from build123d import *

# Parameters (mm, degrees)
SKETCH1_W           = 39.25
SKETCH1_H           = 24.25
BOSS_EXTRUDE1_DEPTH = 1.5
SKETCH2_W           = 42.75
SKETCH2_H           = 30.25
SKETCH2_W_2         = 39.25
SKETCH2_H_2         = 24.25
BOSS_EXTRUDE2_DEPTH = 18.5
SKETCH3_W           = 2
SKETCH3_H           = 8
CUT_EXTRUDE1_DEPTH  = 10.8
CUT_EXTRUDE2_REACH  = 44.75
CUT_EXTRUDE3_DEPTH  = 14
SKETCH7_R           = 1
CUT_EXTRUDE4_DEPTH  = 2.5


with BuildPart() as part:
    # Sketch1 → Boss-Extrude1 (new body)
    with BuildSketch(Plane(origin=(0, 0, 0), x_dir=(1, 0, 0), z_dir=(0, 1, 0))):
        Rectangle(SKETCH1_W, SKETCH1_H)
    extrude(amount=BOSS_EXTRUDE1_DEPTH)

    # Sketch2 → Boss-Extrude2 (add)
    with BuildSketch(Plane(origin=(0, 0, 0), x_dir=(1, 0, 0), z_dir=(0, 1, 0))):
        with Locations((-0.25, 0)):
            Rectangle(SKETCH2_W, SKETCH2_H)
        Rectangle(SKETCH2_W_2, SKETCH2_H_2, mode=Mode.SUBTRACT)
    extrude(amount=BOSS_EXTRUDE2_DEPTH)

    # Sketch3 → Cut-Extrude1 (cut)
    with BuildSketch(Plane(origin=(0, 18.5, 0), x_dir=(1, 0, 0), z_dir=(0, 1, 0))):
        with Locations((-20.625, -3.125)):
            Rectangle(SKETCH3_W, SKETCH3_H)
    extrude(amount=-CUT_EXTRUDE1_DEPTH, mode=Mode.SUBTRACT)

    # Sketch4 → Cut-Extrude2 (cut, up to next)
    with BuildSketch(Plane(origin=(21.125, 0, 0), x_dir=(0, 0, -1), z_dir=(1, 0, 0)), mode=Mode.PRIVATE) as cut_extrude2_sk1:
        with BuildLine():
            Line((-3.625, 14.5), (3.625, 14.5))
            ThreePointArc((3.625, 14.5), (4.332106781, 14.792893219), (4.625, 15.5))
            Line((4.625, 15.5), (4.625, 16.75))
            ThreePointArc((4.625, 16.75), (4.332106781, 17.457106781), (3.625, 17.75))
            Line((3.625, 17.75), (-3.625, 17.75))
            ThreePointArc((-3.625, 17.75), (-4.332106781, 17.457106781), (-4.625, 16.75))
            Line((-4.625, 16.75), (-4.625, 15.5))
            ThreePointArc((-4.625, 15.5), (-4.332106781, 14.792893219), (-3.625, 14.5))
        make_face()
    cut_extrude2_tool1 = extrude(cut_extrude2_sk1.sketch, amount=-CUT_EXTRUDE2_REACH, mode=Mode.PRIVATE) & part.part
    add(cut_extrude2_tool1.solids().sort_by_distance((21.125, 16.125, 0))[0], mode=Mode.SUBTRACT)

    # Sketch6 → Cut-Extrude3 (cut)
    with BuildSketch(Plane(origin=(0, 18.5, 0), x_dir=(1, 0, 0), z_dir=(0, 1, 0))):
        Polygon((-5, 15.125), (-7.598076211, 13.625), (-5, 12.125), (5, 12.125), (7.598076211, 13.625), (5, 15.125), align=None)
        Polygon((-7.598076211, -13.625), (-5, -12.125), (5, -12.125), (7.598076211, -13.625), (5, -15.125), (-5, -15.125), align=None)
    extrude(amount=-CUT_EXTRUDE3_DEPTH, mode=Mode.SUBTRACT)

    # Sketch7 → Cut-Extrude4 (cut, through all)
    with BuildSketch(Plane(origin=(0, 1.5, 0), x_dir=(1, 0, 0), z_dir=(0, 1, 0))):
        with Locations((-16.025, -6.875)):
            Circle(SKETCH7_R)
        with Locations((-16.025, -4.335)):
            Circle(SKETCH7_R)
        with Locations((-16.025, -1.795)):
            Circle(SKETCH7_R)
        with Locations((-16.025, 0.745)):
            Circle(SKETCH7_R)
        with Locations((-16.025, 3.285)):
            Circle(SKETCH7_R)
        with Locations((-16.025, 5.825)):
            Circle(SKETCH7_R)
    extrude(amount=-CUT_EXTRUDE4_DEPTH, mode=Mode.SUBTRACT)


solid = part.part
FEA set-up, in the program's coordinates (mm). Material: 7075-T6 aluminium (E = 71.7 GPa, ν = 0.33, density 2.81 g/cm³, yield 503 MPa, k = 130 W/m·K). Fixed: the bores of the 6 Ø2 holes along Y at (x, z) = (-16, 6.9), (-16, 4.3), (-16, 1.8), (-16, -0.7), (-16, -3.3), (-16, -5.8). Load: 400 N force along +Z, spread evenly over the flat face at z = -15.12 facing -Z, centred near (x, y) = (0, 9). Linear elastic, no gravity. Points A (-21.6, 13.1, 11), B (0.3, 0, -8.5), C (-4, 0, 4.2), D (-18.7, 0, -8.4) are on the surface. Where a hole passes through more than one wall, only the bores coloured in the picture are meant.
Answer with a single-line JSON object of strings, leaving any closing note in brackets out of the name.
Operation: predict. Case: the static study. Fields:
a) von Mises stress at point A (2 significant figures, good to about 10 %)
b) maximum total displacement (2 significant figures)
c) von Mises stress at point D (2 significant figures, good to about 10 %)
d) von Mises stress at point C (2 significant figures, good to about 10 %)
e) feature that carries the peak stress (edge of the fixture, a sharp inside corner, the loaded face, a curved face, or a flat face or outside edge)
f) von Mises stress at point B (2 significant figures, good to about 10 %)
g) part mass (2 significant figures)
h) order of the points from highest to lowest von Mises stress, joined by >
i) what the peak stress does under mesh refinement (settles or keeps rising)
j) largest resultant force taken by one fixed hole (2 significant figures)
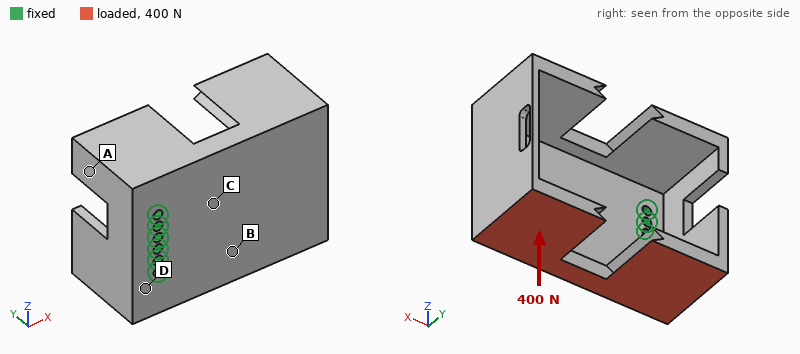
{"von Mises stress at point A": "12 MPa", "maximum total displacement": "0.26 mm", "von Mises stress at point D": "65 MPa", "von Mises stress at point C": "6.3 MPa", "feature that carries the peak stress": "edge of the fixture", "von Mises stress at point B": "24 MPa", "part mass": "18 g", "order of the points from highest to lowest von Mises stress, joined by >": "D > B > A > C", "what the peak stress does under mesh refinement": "keeps rising", "largest resultant force taken by one fixed hole": "460 N"}
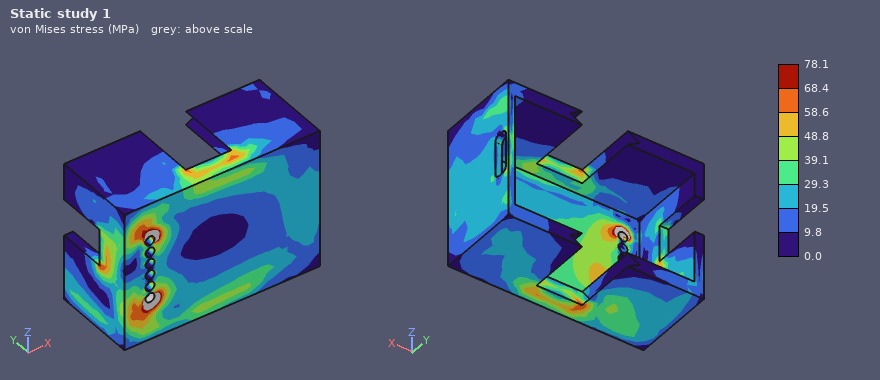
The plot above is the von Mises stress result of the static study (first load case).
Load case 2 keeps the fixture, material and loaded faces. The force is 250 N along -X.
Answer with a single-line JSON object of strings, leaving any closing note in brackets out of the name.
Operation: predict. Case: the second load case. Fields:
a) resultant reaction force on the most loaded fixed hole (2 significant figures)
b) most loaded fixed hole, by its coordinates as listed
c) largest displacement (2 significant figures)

{"resultant reaction force on the most loaded fixed hole": "370 N", "most loaded fixed hole, by its coordinates as listed": "(-16, -5.8)", "largest displacement": "0.37 mm"}
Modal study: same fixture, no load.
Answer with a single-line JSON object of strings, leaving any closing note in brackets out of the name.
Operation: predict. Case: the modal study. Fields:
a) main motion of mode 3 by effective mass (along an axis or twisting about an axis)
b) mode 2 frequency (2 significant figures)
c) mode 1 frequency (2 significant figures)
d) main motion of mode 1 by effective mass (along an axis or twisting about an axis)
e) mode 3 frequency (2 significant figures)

{"main motion of mode 3 by effective mass": "along Z", "mode 2 frequency": "1600 Hz", "mode 1 frequency": "850 Hz", "main motion of mode 1 by effective mass": "along Y", "mode 3 frequency": "4400 Hz"}
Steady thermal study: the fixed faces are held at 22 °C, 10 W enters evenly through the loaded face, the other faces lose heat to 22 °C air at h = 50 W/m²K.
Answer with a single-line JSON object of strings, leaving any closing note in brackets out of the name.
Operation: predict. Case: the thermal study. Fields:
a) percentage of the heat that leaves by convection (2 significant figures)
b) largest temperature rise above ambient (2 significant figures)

{"percentage of the heat that leaves by convection": "30 %", "largest temperature rise above ambient": "22 K"}
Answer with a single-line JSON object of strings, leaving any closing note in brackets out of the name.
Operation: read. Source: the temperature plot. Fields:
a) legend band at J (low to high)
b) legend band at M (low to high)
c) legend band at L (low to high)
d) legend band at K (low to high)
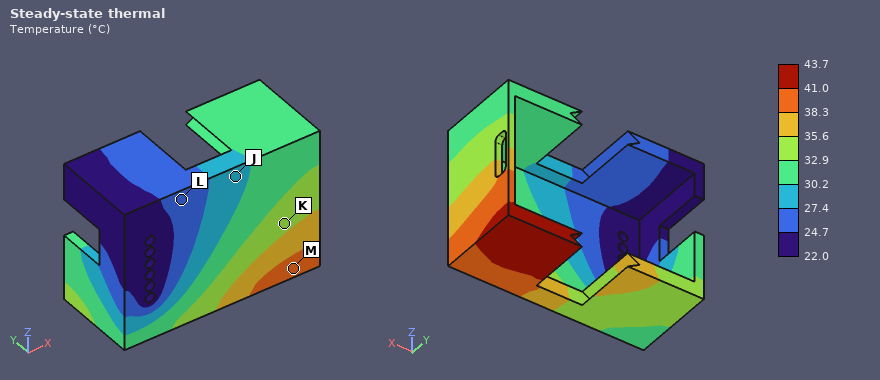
{"legend band at J": "27.4 to 30.2 °C", "legend band at M": "38.3 to 41.0 °C", "legend band at L": "24.7 to 27.4 °C", "legend band at K": "32.9 to 35.6 °C"}
